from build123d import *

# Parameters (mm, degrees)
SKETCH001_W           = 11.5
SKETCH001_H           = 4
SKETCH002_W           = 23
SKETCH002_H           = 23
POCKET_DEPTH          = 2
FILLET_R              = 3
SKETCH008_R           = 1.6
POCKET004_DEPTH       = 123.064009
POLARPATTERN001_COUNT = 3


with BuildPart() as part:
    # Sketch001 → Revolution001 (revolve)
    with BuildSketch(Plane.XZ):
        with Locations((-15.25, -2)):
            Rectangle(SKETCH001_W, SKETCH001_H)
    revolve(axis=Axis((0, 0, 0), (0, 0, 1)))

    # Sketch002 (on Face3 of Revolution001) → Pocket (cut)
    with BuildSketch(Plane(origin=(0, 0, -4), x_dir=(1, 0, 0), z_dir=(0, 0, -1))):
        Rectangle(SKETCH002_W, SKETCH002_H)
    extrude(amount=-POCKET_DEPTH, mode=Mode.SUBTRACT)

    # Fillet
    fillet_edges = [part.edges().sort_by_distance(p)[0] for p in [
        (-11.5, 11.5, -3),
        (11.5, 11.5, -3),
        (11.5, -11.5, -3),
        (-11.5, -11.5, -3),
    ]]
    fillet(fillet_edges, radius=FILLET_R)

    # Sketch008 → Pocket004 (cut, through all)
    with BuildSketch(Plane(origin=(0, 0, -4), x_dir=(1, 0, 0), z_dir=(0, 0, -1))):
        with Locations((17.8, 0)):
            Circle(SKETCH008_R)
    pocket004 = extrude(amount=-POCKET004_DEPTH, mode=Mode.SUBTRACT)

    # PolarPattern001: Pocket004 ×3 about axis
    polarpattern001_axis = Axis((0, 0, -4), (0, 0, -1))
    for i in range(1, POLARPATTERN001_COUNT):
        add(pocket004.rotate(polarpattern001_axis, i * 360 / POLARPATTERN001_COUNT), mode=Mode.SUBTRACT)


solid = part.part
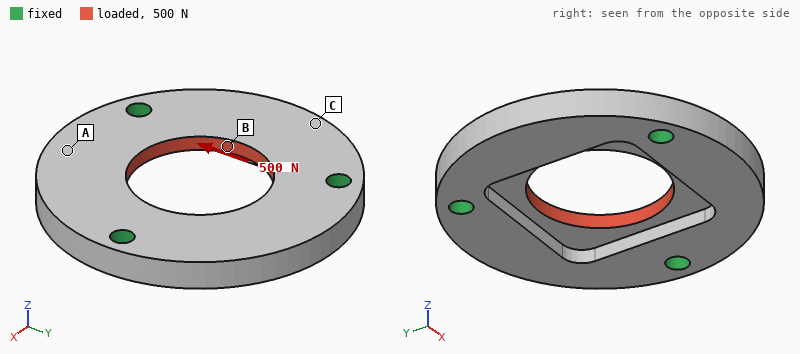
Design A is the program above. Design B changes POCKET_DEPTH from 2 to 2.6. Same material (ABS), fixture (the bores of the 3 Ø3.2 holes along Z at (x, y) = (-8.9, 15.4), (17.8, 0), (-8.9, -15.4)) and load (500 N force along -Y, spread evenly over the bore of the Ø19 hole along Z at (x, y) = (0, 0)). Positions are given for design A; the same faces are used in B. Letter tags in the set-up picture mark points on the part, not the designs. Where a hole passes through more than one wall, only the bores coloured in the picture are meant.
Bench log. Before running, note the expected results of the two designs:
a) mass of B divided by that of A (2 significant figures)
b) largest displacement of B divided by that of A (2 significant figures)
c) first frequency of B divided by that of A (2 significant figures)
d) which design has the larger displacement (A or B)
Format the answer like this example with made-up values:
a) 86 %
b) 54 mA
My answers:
a) 0.96
b) 1.3
c) 1.00
d) B
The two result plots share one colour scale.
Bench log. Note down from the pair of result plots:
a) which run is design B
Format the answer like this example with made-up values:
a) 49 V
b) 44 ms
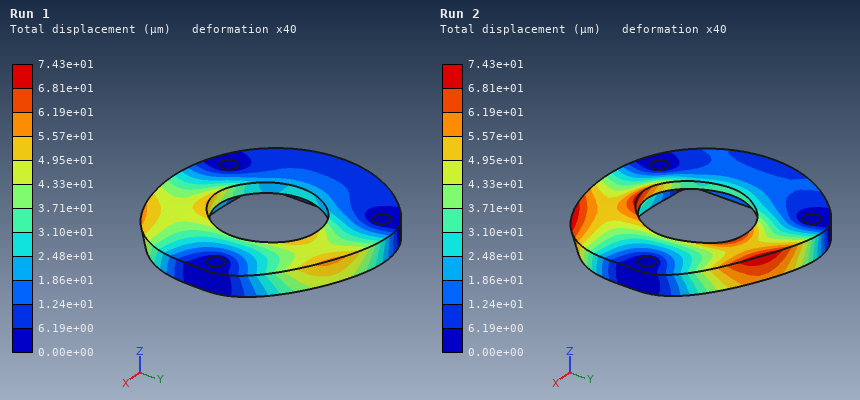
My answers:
a) Run 2
